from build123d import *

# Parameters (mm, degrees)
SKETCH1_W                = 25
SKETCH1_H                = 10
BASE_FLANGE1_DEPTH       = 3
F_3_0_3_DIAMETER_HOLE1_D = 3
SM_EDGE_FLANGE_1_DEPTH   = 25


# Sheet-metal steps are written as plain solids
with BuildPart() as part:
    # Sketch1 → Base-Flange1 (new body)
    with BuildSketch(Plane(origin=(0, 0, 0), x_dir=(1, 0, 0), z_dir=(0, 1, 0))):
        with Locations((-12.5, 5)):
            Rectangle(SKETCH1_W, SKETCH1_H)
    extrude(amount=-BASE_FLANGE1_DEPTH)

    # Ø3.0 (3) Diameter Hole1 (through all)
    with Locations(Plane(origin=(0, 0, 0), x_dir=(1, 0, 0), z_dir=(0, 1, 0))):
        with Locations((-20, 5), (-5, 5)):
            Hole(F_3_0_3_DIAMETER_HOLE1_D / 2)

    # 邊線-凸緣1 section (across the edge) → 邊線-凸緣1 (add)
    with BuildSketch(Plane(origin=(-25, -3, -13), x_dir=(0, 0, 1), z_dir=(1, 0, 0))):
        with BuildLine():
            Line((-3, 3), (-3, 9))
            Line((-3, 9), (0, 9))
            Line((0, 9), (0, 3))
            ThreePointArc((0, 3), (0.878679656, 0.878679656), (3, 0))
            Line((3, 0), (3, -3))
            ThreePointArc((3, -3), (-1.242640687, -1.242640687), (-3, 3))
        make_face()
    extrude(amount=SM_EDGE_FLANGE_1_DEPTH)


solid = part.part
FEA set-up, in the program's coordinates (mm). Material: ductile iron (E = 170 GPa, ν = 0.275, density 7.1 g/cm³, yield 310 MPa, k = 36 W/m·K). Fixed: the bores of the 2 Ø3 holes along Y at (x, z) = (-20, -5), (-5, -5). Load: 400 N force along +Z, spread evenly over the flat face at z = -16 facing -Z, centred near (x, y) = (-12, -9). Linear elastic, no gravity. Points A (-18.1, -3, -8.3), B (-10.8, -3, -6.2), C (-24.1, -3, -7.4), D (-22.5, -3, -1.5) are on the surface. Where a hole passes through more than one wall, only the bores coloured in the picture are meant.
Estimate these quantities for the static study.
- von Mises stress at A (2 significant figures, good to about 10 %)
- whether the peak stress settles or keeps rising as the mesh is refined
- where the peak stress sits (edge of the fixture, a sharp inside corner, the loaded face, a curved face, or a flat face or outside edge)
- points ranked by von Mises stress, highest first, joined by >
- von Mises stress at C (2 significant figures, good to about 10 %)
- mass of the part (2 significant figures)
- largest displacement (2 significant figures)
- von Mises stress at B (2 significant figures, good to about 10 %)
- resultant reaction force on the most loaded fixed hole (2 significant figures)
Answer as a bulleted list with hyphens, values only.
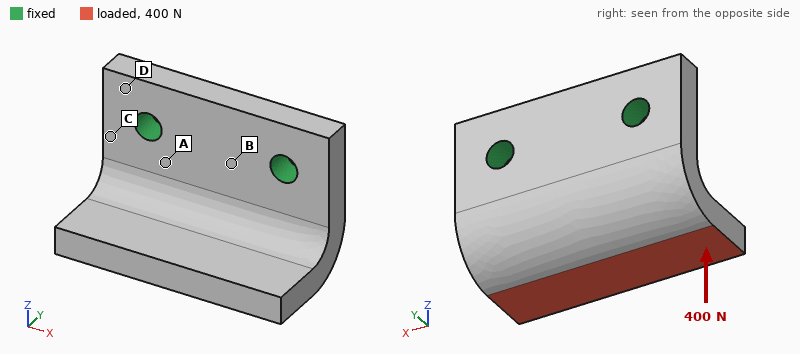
- 84 MPa
- keeps rising
- edge of the fixture
- A > C > B > D
- 67 MPa
- 12 g
- 37 µm
- 45 MPa
- 200 N
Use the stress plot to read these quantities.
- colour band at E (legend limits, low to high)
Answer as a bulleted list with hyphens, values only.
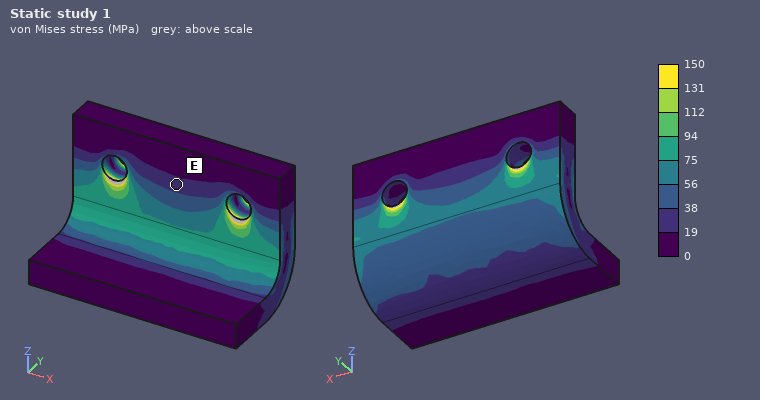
- 19 to 38 MPa
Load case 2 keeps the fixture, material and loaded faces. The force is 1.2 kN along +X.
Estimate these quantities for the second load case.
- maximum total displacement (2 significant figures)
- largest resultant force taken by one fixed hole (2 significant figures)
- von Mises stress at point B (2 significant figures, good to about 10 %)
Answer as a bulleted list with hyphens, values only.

- 27 µm
- 1.1 kN
- 53 MPa
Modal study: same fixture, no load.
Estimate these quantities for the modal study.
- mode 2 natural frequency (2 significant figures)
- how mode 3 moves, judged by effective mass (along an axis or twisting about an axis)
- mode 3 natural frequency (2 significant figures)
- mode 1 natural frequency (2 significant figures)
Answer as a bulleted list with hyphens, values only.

- 14 kHz
- along Y
- 26 kHz
- 8600 Hz
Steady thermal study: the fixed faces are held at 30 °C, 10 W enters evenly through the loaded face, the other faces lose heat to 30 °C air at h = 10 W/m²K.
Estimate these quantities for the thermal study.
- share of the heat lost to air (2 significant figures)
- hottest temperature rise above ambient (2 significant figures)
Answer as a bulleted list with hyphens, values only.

- 3.0 %
- 57 K
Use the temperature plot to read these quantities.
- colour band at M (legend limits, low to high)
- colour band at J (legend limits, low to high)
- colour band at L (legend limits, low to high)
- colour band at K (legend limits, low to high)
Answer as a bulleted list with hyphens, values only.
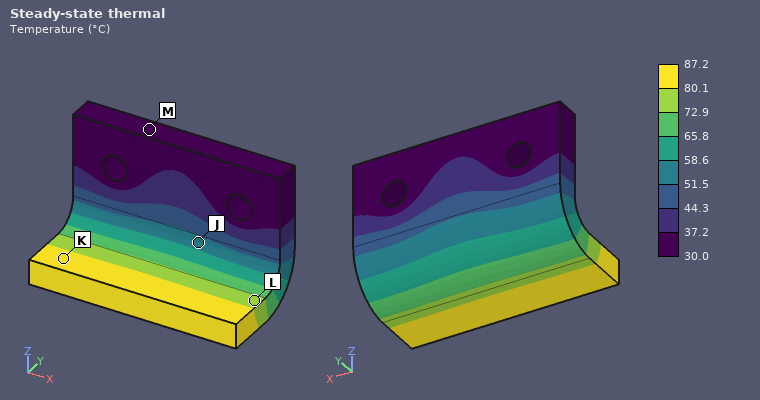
- 30.0 to 37.2 °C
- 51.5 to 58.6 °C
- 72.9 to 80.1 °C
- 80.1 to 87.2 °C
